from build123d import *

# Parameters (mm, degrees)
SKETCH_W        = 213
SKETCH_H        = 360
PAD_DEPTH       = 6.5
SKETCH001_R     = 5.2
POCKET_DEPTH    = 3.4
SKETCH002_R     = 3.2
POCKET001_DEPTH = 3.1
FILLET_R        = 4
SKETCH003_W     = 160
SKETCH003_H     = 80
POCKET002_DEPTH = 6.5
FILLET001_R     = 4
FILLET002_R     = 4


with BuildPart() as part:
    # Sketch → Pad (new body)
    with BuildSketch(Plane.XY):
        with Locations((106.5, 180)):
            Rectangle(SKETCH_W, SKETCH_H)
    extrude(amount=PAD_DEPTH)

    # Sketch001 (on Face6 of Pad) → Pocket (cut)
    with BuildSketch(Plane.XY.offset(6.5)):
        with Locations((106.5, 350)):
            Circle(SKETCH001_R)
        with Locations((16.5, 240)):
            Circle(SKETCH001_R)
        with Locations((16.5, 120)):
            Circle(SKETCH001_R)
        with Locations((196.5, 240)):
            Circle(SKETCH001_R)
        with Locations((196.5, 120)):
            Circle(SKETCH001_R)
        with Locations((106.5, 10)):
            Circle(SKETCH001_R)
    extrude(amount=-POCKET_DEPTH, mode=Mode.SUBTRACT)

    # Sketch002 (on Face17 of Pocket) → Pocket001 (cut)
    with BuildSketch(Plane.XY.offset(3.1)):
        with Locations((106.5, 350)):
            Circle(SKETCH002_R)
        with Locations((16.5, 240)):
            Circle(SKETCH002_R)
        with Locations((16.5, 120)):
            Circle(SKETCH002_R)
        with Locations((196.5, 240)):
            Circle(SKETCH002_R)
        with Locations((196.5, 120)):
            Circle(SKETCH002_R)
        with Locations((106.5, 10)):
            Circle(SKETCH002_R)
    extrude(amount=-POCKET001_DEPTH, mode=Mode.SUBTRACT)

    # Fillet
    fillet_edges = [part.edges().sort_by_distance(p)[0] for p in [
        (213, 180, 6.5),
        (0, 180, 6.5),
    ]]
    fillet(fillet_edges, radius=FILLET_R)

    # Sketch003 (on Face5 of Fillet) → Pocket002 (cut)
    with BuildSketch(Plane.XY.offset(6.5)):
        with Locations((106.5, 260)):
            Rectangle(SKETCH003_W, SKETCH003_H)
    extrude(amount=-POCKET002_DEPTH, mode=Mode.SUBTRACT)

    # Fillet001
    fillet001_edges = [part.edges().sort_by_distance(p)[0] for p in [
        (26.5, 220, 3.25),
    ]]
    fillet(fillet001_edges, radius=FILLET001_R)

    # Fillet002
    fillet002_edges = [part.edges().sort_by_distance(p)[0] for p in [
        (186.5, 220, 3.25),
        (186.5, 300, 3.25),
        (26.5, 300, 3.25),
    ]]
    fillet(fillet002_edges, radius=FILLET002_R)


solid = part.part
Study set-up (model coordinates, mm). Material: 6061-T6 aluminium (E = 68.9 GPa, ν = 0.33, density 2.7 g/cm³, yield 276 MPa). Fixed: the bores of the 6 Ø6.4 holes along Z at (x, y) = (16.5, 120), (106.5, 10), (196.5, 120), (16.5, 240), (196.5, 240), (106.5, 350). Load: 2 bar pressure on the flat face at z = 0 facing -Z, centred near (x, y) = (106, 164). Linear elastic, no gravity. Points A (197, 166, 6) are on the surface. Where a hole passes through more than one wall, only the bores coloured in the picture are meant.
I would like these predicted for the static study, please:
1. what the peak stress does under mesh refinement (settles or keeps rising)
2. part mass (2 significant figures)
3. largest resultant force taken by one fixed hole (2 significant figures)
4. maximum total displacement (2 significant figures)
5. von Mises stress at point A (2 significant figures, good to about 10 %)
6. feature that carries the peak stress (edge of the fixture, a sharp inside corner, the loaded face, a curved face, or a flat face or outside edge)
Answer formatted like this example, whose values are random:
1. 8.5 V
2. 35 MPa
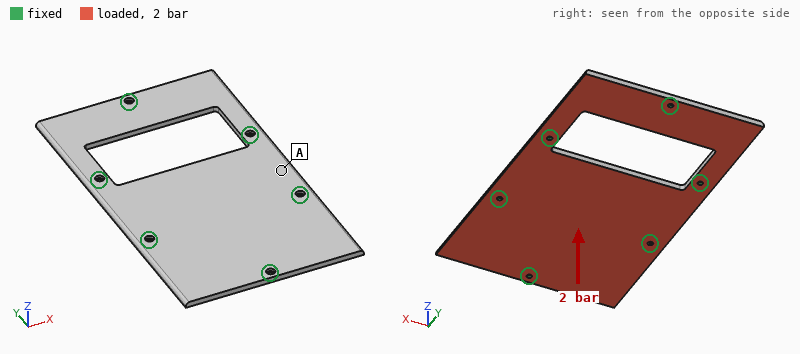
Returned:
1. keeps rising
2. 1.1 kg
3. 4.1 kN
4. 1.1 mm
5. 20 MPa
6. edge of the fixture
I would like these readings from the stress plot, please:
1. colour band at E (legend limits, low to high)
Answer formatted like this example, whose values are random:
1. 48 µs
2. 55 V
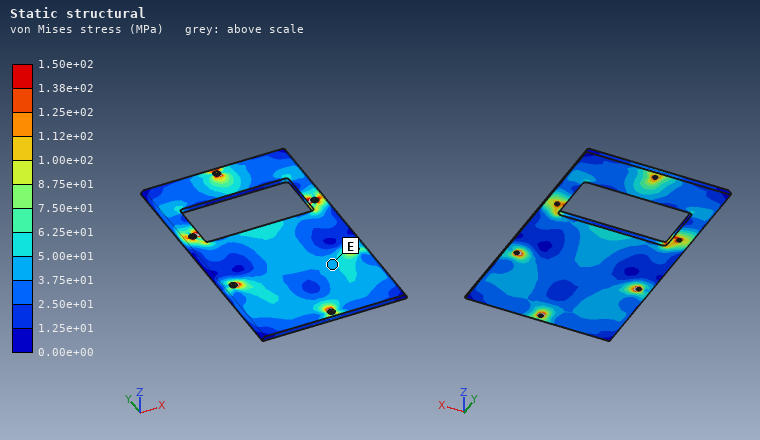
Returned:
1. 3.75e+01 to 5.00e+01 MPa
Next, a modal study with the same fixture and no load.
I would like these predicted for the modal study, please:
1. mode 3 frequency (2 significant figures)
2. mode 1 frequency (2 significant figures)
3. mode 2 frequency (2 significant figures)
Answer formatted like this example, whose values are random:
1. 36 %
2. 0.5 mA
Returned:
1. 680 Hz
2. 570 Hz
3. 670 Hz
